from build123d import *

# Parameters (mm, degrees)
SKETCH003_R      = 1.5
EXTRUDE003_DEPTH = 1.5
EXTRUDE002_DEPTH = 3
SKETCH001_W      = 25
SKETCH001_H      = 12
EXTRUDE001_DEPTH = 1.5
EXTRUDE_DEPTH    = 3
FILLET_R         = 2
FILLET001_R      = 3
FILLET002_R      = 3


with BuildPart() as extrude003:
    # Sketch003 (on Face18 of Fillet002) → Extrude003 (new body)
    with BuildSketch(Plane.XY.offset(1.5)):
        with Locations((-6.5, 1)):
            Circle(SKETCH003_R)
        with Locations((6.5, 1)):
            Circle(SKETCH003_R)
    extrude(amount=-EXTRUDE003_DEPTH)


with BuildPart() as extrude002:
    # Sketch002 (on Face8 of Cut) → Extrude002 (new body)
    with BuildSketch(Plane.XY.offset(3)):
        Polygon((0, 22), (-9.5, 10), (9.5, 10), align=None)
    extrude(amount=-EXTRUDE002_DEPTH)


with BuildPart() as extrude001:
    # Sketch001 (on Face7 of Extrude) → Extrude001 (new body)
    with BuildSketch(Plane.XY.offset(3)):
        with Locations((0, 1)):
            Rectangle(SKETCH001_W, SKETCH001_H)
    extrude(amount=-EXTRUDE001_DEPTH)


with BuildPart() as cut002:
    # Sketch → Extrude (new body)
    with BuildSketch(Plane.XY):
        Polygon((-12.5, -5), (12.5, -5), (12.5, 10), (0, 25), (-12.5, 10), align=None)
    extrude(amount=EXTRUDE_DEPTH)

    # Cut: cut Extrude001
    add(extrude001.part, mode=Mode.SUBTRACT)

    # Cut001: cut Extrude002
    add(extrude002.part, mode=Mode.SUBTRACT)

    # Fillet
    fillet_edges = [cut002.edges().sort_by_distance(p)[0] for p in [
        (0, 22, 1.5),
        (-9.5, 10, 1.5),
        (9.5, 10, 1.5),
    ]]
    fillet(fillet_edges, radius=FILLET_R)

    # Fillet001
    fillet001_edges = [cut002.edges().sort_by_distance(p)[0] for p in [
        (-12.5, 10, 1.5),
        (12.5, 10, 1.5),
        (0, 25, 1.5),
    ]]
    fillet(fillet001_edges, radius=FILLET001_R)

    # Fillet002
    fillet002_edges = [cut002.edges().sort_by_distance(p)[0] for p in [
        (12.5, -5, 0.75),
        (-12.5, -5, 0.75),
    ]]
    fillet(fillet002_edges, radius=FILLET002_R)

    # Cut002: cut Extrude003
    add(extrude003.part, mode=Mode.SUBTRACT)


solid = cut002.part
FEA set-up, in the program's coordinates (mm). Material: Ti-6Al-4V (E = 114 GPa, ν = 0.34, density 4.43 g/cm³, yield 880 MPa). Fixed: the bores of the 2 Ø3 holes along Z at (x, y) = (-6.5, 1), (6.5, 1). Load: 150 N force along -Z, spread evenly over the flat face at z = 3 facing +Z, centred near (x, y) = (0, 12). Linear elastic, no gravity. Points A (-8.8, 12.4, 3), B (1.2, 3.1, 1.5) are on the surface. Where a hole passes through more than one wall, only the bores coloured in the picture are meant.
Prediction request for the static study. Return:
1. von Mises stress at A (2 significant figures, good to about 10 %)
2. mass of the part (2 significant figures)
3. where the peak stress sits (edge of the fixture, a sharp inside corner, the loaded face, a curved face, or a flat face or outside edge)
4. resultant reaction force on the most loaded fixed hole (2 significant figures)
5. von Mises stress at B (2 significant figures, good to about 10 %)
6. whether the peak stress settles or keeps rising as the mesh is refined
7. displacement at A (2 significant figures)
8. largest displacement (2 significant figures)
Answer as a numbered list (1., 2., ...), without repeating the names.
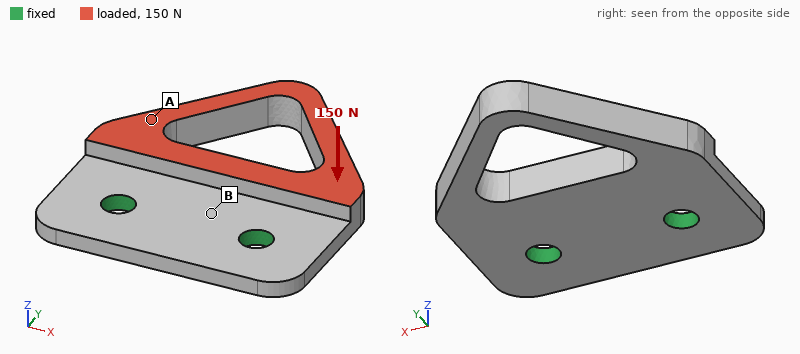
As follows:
1. 38 MPa
2. 3.9 g
3. edge of the fixture
4. 75 N
5. 87 MPa
6. keeps rising
7. 0.075 mm
8. 0.19 mm
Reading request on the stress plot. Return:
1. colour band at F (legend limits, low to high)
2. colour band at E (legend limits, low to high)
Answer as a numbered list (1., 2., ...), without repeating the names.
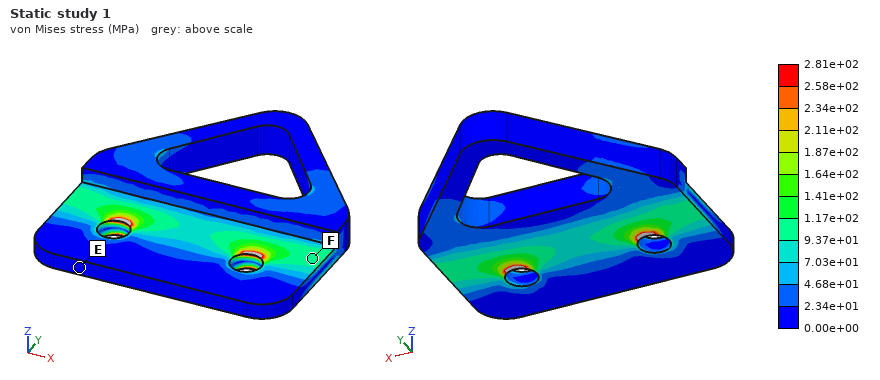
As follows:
1. 9.37e+01 to 1.17e+02 MPa
2. 0.00e+00 to 2.34e+01 MPa
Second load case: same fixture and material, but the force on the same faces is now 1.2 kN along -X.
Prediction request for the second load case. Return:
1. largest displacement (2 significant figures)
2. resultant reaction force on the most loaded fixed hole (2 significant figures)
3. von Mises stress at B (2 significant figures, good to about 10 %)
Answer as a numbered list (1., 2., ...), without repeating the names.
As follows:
1. 60 µm
2. 1.0 kN
3. 110 MPa
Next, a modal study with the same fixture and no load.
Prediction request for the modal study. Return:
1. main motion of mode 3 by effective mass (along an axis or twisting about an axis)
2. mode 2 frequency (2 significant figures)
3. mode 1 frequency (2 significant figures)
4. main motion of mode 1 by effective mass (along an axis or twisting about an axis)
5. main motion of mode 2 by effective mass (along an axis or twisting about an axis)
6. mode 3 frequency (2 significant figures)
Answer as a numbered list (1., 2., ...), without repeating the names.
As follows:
1. along Z
2. 12 kHz
3. 4100 Hz
4. along Z
5. twisting about Y
6. 18 kHz
